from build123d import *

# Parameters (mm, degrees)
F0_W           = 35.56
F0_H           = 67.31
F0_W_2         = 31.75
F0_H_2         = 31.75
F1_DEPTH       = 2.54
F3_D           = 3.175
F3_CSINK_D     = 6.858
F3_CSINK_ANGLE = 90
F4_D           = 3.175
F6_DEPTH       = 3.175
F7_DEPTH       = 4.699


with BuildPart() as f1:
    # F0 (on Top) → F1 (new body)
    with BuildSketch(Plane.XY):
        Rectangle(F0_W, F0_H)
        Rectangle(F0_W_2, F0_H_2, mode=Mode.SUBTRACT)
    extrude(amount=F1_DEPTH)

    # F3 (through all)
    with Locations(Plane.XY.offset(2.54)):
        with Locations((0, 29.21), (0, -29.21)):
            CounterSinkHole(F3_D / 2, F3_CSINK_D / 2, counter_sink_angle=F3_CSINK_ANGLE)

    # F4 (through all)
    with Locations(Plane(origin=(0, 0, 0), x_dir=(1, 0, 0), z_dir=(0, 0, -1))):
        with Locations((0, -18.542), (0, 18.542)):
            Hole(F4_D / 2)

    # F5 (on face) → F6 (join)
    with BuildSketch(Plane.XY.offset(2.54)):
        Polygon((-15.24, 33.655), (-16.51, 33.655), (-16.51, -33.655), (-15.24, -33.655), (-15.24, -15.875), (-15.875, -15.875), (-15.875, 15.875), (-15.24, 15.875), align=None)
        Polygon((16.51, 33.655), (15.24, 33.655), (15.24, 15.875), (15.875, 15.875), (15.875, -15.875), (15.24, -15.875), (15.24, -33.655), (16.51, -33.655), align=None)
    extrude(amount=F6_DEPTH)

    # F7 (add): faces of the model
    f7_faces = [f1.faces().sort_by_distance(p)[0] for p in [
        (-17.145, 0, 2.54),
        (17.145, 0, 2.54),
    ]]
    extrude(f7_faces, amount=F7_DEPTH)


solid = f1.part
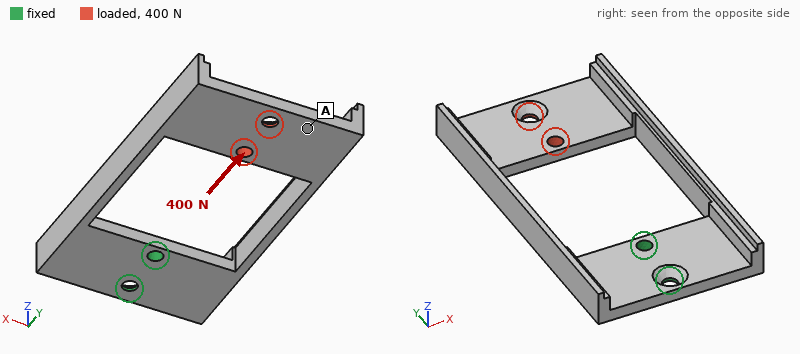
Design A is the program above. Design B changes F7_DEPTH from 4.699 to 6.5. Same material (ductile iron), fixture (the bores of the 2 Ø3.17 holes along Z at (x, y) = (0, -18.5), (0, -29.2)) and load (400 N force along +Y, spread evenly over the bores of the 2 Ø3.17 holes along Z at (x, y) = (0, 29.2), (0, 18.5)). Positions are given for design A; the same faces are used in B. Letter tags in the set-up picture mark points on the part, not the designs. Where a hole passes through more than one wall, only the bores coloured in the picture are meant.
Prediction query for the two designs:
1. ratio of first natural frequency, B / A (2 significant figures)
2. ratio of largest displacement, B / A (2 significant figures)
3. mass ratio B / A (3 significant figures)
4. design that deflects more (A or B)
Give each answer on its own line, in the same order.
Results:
1.1
0.75
1.07
A
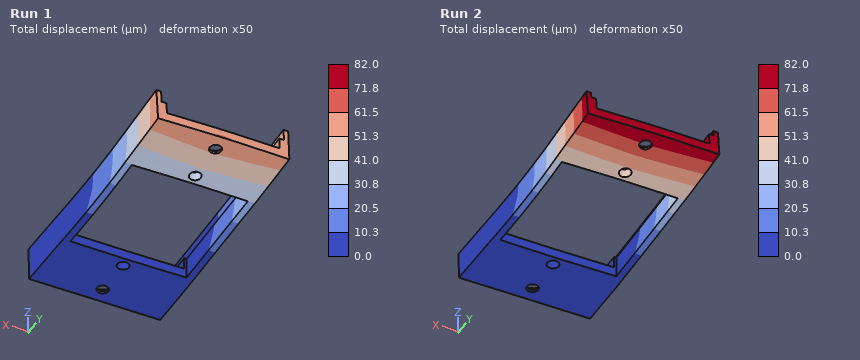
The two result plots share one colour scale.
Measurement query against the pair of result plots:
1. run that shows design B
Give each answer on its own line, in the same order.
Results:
Run 1
